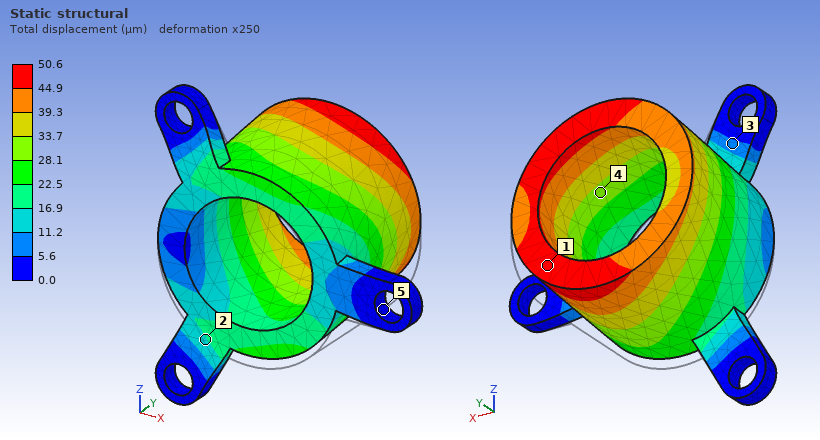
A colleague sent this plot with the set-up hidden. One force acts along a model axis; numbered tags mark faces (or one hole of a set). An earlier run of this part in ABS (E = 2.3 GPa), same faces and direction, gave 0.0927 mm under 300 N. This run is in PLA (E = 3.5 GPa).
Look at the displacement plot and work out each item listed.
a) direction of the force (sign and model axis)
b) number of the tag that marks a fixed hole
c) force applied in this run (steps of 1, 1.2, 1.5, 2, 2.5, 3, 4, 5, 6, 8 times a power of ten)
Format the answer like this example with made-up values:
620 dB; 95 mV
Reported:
+Z; 5; 250 N
